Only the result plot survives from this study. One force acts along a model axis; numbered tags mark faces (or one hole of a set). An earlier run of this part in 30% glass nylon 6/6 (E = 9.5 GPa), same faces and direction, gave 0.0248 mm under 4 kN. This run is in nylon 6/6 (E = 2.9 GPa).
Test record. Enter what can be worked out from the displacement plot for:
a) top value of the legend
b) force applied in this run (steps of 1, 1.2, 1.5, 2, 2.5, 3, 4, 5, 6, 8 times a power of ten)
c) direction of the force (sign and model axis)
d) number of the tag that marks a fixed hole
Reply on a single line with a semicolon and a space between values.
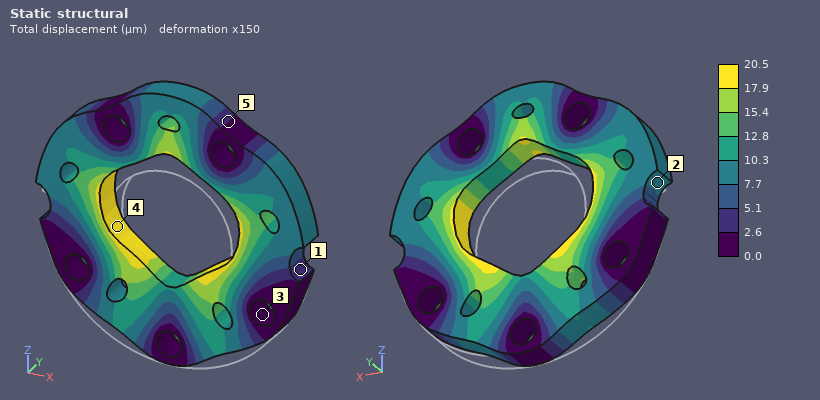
20.5 µm; 1 kN; +Z; 3
